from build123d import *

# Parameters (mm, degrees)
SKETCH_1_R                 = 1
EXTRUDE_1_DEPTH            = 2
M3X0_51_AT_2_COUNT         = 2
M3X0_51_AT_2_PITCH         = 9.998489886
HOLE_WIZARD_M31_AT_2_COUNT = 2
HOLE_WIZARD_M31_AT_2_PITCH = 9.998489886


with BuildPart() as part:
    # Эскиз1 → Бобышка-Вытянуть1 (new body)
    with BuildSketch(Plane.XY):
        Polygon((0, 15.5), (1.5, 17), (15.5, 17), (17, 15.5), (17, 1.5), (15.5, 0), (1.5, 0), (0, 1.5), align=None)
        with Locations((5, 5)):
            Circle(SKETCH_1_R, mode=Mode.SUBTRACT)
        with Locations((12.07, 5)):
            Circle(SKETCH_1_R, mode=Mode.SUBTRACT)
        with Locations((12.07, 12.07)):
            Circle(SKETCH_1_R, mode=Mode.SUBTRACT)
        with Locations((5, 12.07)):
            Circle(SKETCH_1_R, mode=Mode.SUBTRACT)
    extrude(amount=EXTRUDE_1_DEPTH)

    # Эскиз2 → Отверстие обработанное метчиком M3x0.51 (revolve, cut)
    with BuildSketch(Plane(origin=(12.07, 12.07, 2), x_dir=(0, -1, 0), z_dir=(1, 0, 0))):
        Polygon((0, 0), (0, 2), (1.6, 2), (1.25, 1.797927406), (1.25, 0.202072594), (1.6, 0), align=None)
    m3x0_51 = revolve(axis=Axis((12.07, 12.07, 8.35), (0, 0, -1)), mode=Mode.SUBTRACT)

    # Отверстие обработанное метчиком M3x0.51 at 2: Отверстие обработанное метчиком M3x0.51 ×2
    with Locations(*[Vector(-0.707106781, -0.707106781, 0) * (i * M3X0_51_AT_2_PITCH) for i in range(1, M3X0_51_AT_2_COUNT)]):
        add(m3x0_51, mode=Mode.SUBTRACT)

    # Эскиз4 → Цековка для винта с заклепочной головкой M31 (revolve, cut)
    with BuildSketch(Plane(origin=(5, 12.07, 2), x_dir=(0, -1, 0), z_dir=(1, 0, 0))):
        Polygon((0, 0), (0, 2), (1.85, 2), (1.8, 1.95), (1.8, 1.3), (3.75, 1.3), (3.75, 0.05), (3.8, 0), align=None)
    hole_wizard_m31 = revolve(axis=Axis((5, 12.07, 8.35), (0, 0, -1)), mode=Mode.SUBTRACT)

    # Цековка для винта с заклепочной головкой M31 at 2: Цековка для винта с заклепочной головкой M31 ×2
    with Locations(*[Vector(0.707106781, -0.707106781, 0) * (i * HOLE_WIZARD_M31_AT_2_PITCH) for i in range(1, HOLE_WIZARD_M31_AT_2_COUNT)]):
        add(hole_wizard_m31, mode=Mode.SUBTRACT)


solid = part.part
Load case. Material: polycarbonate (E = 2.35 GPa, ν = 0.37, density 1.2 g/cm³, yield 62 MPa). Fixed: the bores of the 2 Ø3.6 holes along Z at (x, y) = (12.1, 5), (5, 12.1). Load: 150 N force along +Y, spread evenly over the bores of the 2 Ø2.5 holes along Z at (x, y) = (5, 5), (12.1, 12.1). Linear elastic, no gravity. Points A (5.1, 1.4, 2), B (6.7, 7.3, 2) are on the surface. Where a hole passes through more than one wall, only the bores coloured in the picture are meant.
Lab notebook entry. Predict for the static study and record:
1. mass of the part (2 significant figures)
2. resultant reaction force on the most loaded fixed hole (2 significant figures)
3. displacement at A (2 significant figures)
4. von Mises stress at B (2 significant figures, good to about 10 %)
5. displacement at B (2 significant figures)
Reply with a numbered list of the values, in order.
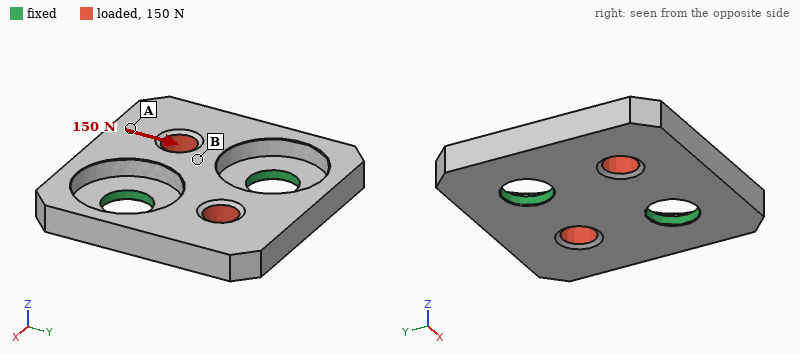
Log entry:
1. 0.50 g
2. 75 N
3. 0.13 mm
4. 8.2 MPa
5. 0.051 mm
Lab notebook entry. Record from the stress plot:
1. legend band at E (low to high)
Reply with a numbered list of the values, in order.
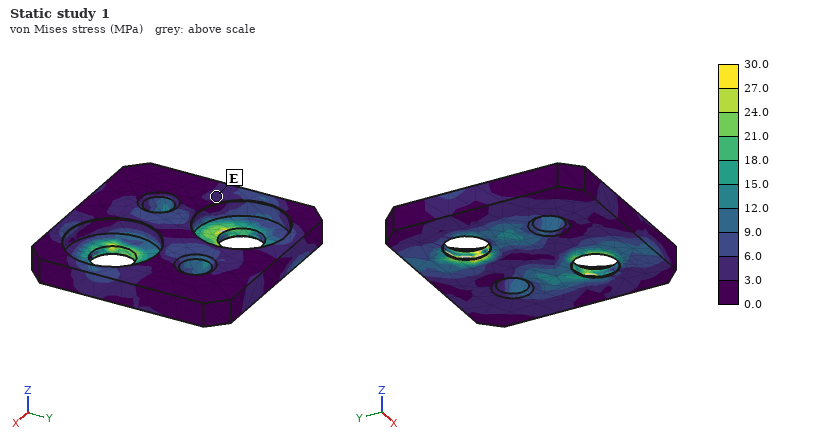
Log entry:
1. 3.0 to 6.0 MPa
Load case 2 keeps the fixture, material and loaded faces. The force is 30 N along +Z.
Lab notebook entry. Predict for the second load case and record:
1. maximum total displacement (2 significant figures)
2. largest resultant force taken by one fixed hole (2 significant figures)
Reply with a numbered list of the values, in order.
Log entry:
1. 0.16 mm
2. 19 N
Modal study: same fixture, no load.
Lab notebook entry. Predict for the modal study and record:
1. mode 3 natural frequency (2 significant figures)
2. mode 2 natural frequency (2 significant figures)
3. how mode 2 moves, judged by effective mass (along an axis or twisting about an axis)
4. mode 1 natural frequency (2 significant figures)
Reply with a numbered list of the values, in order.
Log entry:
1. 9600 Hz
2. 4200 Hz
3. along Z
4. 3000 Hz
